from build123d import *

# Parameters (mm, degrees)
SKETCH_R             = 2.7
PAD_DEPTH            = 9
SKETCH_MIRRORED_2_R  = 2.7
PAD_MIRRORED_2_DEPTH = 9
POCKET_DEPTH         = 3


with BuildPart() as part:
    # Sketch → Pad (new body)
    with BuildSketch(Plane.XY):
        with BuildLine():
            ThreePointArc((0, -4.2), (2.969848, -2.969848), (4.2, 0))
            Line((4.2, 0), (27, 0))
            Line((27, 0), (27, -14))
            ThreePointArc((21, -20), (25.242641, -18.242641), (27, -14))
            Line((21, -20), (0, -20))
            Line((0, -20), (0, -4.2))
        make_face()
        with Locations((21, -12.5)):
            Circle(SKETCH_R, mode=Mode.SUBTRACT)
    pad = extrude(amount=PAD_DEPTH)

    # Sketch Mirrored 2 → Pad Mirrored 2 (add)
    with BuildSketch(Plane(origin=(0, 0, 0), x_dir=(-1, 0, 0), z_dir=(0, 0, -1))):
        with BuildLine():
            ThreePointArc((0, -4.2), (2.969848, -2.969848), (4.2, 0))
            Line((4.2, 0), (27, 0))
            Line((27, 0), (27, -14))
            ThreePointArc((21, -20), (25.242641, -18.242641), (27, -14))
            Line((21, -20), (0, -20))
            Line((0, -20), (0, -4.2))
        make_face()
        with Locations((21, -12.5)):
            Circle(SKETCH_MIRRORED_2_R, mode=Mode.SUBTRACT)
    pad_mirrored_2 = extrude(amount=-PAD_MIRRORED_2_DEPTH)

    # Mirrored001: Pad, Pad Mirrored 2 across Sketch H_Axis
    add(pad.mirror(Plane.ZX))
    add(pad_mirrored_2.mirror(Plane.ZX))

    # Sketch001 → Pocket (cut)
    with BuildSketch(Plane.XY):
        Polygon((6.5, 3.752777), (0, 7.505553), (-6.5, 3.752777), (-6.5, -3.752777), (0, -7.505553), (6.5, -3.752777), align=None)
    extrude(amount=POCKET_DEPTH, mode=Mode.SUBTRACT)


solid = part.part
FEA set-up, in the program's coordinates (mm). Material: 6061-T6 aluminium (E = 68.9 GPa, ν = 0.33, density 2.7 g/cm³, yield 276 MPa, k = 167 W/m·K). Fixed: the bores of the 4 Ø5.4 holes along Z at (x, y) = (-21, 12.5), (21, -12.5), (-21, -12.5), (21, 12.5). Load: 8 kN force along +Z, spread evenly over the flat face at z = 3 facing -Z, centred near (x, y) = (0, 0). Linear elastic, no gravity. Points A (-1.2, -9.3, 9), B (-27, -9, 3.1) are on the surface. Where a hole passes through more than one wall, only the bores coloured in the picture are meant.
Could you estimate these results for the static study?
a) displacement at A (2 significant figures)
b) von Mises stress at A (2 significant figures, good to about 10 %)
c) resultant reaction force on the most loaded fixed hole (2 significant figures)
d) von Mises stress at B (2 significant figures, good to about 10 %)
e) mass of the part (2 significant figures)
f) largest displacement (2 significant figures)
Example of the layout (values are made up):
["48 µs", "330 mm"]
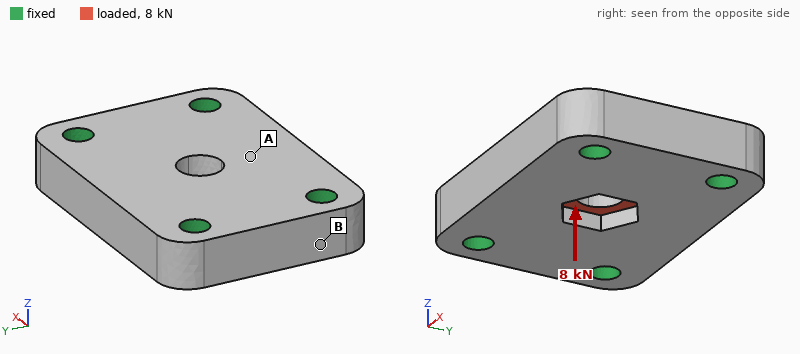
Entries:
["33 µm", "79 MPa", "2.0 kN", "28 MPa", "47 g", "50 µm"]
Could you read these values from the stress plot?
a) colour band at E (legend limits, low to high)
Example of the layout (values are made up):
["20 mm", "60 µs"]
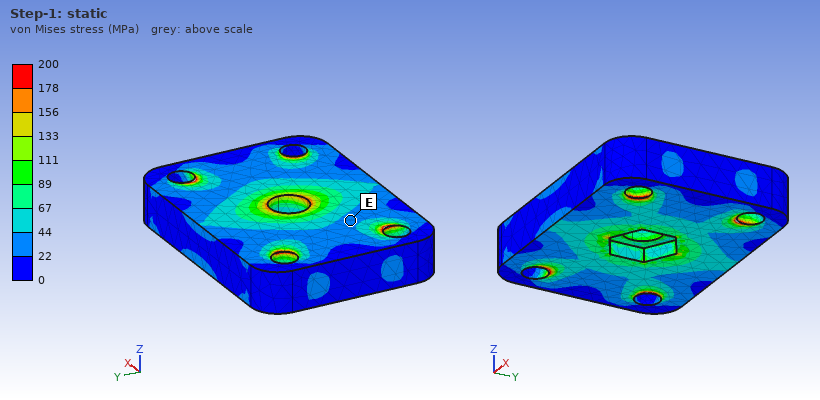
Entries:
["22 to 44 MPa"]
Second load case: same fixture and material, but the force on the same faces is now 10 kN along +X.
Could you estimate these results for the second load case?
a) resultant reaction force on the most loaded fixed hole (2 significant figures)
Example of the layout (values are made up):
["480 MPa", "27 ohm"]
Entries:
["2.7 kN"]
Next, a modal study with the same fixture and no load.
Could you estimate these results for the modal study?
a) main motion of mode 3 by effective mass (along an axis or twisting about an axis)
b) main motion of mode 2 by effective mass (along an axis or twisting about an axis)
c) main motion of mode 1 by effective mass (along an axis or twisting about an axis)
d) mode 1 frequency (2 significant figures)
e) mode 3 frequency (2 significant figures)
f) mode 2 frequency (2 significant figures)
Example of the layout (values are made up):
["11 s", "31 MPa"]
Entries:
["along Y", "twisting about X", "along Z", "21 kHz", "34 kHz", "25 kHz"]
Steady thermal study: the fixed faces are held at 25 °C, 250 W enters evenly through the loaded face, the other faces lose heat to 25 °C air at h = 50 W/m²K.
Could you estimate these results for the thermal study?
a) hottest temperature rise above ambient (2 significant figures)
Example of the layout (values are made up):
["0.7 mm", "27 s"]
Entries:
["78 K"]
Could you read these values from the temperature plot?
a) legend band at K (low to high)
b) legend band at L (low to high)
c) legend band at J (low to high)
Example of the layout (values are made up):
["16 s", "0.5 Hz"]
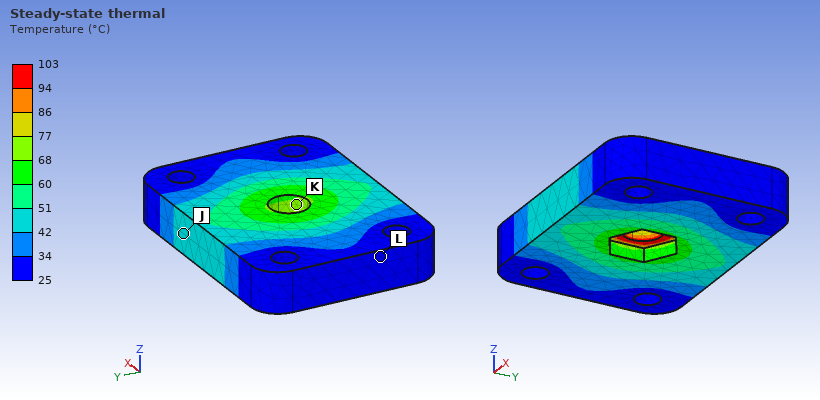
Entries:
["68 to 77 °C", "25 to 34 °C", "42 to 51 °C"]
